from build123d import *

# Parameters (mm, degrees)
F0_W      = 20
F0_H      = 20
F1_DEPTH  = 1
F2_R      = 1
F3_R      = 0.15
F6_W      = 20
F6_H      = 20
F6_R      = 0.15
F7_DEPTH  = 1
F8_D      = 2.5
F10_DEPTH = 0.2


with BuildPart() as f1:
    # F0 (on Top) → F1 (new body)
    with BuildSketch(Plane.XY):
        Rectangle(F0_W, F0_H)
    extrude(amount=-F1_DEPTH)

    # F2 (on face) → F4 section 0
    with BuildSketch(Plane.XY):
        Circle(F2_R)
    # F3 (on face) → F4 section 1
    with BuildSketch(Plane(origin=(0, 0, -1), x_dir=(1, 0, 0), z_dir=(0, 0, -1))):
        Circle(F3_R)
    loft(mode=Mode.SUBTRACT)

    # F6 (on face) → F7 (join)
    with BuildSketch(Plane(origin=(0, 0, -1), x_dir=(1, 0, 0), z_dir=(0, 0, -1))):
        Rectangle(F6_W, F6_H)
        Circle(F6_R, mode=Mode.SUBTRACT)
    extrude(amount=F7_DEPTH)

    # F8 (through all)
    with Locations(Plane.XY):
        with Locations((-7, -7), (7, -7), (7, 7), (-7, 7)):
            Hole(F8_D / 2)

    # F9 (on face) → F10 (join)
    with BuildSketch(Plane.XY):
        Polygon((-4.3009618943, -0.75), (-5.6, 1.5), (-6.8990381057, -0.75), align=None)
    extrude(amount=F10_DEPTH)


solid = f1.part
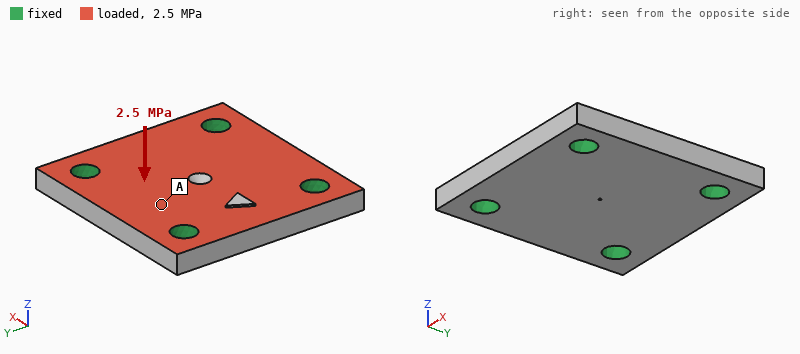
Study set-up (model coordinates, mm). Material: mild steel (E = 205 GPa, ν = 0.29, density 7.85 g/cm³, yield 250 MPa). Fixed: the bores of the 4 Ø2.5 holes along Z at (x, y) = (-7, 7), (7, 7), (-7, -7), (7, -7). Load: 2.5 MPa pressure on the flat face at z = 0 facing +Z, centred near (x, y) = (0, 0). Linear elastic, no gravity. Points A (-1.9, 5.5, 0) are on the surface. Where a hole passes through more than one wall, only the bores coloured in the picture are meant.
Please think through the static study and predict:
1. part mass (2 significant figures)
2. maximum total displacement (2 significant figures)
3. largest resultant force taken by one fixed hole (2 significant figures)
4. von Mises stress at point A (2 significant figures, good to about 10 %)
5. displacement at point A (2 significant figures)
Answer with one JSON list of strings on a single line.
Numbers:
["6.0 g", "3.5 µm", "240 N", "21 MPa", "2.0 µm"]
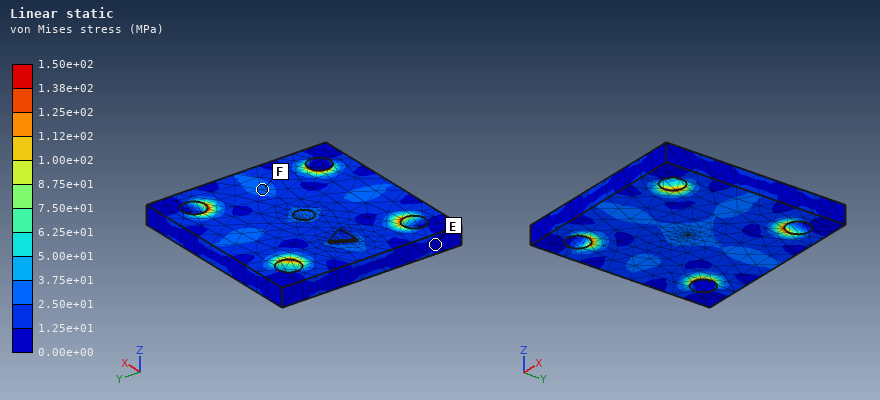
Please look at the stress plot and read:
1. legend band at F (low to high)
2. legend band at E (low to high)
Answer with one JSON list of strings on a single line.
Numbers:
["2.50e+01 to 3.75e+01 MPa", "0.00e+00 to 1.25e+01 MPa"]
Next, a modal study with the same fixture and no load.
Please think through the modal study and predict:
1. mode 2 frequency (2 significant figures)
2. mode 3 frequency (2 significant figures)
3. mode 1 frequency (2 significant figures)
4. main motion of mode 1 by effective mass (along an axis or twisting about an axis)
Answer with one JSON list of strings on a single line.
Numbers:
["60 kHz", "60 kHz", "41 kHz", "along Z"]
